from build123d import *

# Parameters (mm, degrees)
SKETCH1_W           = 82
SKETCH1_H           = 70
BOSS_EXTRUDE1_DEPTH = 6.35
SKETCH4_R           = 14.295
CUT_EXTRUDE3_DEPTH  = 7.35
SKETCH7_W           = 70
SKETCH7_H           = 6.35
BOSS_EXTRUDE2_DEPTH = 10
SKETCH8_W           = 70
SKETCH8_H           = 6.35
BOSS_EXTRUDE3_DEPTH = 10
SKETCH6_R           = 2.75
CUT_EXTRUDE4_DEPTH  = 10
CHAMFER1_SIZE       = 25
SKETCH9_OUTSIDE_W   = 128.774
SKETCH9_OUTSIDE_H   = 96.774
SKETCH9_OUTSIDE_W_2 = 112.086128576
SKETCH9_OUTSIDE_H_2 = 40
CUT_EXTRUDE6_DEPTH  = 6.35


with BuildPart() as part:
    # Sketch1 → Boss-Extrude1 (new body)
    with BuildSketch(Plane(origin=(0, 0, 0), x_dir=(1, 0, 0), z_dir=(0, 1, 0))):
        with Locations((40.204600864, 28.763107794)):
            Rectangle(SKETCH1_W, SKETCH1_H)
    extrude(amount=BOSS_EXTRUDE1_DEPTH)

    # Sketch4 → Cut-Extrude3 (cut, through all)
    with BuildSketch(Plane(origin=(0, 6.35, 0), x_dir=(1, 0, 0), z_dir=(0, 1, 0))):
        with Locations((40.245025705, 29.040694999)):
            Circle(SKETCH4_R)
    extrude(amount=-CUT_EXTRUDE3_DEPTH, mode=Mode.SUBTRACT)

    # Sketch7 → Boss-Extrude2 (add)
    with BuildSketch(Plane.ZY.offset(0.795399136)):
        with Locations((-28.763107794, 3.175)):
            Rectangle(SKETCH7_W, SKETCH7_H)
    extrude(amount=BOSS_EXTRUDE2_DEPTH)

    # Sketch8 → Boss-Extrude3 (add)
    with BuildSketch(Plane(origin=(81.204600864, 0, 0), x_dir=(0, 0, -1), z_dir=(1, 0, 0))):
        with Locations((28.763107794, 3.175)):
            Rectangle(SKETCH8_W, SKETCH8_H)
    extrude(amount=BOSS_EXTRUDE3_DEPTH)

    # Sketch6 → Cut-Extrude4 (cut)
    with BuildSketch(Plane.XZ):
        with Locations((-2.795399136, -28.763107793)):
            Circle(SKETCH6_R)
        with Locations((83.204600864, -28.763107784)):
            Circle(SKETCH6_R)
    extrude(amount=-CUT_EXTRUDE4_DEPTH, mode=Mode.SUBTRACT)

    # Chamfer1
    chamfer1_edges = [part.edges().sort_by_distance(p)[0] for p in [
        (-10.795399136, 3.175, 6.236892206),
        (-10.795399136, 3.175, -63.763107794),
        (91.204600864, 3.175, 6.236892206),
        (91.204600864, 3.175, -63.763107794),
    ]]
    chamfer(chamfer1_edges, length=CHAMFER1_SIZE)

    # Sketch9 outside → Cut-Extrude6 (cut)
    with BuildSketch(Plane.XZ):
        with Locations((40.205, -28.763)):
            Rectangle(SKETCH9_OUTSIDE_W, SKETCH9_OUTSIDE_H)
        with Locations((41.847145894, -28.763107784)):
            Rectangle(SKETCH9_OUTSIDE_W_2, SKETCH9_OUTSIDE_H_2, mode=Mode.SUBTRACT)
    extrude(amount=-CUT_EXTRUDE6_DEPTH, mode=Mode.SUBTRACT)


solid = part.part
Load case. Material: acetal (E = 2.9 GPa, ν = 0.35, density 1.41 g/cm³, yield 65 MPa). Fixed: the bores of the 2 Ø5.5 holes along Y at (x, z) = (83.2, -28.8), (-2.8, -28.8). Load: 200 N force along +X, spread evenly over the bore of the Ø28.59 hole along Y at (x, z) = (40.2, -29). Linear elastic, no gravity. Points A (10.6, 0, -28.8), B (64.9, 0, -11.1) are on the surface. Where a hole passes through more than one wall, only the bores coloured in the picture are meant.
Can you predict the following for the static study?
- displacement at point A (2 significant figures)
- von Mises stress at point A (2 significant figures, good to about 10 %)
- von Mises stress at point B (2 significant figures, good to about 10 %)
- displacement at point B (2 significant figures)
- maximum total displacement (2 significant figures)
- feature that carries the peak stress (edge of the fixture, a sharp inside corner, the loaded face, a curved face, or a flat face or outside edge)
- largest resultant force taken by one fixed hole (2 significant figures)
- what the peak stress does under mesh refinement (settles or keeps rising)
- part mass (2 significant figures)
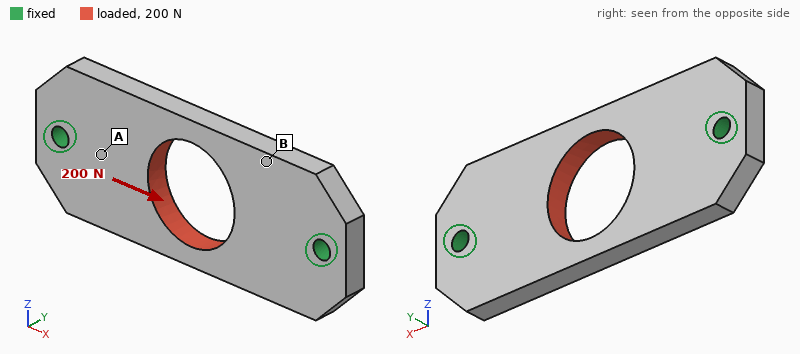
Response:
3.5 µm
0.68 MPa
0.30 MPa
5.6 µm
9.3 µm
edge of the fixture
100 N
keeps rising
29 g
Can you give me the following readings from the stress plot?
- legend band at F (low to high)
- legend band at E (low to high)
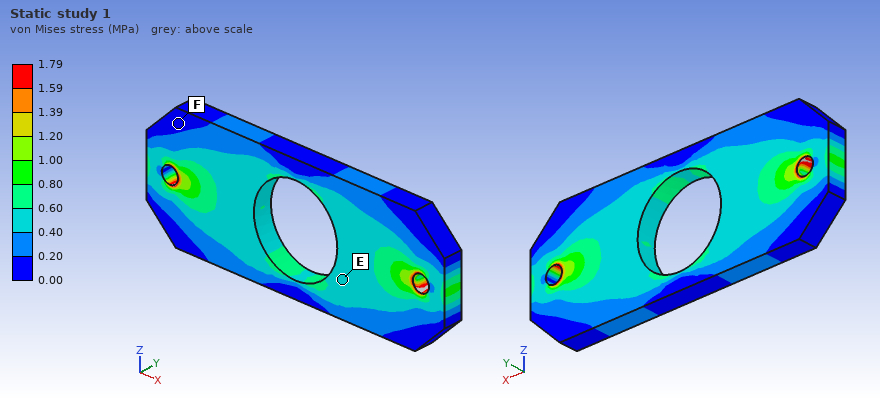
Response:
0.00 to 0.20 MPa
0.40 to 0.60 MPa
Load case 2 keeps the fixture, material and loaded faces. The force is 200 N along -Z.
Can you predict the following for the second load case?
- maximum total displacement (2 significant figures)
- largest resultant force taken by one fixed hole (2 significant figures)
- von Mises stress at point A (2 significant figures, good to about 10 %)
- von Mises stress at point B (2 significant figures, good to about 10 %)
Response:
42 µm
100 N
1.0 MPa
0.71 MPa
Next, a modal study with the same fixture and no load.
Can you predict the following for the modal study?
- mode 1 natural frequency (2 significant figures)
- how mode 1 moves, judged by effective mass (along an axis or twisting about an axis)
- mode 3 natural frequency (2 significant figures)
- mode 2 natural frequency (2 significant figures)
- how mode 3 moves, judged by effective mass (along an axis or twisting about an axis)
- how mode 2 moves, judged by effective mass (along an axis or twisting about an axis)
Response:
1200 Hz
along Y
2600 Hz
1500 Hz
twisting about Z
twisting about X
